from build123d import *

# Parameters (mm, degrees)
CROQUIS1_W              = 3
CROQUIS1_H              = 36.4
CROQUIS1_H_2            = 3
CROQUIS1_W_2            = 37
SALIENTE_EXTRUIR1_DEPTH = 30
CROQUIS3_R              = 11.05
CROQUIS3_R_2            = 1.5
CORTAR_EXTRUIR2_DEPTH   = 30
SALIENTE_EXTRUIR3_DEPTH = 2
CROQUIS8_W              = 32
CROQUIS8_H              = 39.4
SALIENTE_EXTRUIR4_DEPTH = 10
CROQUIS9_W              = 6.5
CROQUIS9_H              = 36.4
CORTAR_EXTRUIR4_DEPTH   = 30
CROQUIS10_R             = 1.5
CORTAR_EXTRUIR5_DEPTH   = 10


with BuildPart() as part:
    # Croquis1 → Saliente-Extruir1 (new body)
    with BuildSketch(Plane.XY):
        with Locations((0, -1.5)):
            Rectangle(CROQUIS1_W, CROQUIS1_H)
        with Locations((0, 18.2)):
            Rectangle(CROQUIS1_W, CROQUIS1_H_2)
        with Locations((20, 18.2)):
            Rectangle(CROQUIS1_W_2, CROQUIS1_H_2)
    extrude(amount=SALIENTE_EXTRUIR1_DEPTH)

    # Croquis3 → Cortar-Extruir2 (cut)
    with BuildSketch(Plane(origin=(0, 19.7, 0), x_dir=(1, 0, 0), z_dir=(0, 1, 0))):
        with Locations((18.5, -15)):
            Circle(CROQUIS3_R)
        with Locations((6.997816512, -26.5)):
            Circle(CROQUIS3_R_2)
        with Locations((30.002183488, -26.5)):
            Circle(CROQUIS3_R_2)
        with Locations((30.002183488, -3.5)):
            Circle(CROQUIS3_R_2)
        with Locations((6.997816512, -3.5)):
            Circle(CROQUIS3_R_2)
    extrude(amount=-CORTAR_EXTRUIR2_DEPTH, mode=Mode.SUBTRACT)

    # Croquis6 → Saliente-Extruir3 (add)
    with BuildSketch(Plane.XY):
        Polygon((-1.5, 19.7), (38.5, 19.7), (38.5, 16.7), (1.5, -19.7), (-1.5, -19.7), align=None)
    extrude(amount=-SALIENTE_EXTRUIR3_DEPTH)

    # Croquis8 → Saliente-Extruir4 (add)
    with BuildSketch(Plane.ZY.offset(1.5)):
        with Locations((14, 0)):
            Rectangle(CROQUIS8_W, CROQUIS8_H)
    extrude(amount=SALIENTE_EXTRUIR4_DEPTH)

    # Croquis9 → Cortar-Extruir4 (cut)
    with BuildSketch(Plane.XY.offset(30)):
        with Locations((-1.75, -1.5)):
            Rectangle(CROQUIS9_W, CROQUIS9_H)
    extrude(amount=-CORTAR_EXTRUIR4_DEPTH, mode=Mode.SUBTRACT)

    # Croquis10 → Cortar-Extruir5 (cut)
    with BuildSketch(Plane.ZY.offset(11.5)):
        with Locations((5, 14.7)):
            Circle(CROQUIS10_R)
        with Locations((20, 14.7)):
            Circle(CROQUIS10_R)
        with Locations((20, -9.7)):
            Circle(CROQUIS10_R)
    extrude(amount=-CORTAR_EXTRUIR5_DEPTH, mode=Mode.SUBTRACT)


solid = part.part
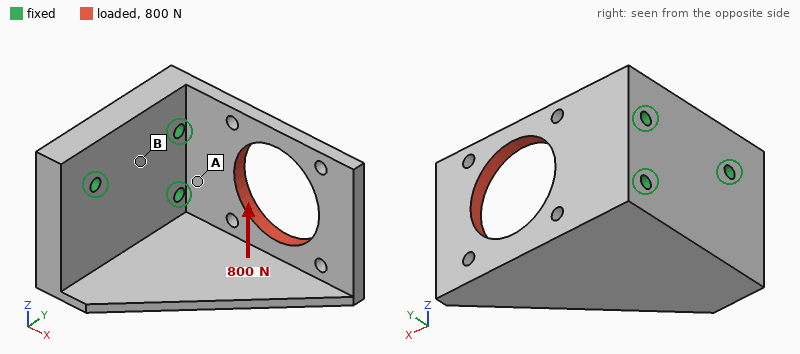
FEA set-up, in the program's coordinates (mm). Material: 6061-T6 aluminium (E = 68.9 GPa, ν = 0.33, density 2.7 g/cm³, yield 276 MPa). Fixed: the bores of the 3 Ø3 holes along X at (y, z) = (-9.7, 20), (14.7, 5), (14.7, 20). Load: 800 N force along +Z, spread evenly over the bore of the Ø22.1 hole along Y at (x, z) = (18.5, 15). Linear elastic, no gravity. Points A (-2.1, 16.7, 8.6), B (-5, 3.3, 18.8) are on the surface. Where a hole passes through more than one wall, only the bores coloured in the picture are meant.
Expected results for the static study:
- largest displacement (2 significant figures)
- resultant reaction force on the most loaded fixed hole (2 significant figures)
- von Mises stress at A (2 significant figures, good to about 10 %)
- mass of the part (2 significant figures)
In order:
91 µm
1.1 kN
30 MPa
35 g
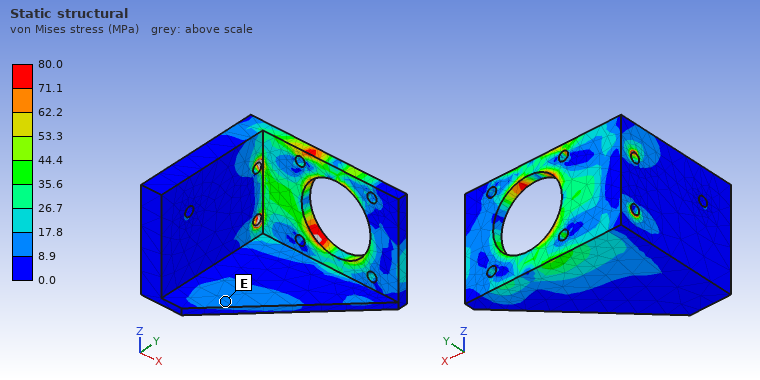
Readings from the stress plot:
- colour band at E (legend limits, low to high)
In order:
8.9 to 17.8 MPa
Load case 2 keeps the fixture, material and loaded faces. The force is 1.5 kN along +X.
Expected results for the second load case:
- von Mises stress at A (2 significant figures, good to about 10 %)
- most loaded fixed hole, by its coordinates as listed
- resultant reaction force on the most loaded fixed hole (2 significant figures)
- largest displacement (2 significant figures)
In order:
12 MPa
(14.7, 20)
970 N
37 µm
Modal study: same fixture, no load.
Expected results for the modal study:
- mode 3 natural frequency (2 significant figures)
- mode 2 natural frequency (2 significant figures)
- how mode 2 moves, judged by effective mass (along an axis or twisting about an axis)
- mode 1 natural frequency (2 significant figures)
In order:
5900 Hz
5100 Hz
along Z
2200 Hz
